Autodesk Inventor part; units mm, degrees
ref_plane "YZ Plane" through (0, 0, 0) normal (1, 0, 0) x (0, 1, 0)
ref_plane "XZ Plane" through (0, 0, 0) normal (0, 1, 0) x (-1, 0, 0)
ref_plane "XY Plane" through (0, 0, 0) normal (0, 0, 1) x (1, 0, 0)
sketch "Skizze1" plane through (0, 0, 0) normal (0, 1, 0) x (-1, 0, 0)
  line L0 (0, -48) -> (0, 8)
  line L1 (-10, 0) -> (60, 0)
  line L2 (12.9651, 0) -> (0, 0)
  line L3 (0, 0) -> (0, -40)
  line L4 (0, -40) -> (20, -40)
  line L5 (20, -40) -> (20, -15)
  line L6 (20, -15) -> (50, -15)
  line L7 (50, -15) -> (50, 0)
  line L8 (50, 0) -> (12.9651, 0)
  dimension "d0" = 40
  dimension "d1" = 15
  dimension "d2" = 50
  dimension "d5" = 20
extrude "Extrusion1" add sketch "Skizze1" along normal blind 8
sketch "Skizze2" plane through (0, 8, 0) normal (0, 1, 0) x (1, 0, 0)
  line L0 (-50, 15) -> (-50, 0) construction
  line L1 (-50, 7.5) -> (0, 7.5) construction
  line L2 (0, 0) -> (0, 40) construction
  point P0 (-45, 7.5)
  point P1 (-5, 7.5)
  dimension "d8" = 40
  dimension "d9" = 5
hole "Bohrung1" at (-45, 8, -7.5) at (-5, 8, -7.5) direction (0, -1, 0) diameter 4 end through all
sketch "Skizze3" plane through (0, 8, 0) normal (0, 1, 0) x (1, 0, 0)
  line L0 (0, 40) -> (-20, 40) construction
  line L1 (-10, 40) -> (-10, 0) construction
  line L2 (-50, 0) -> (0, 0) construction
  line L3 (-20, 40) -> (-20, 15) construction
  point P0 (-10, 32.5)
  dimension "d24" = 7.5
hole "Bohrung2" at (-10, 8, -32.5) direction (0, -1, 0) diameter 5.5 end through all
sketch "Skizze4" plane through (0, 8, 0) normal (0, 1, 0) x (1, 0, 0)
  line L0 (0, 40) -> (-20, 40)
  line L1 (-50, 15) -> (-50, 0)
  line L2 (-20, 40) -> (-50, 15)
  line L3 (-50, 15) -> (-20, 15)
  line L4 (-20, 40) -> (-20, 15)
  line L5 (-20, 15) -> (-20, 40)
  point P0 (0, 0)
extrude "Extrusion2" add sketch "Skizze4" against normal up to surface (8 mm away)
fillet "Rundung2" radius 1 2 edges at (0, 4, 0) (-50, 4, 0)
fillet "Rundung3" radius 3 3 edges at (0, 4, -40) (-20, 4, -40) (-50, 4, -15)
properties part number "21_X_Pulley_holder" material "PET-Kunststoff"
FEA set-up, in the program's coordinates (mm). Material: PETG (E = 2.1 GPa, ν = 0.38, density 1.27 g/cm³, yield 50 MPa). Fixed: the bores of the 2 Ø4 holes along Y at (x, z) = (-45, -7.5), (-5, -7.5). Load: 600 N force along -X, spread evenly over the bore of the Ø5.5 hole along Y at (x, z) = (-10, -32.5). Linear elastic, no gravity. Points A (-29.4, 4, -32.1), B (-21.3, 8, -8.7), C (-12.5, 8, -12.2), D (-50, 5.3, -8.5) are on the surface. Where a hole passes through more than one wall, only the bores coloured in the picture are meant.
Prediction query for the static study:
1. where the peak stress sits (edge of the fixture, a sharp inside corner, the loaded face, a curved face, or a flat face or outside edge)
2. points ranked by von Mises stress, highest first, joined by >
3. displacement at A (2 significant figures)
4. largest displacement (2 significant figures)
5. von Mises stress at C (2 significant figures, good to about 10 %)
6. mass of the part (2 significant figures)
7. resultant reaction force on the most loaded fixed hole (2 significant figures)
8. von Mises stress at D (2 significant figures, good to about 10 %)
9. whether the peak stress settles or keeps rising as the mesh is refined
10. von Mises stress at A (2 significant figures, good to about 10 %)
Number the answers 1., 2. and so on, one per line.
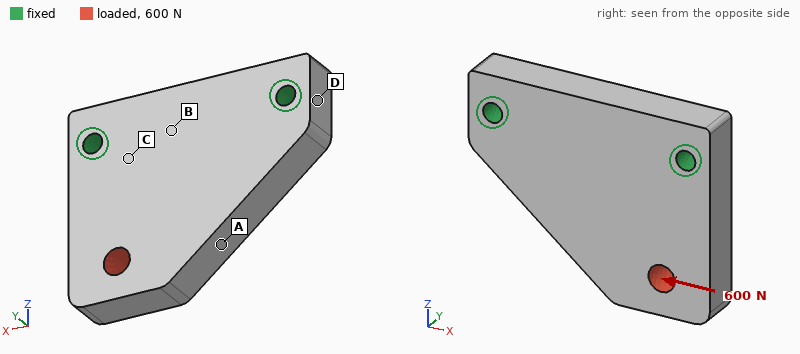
1. edge of the fixture
2. A > D > C > B
3. 0.083 mm
4. 0.14 mm
5. 2.6 MPa
6. 16 g
7. 500 N
8. 4.1 MPa
9. keeps rising
10. 5.4 MPa
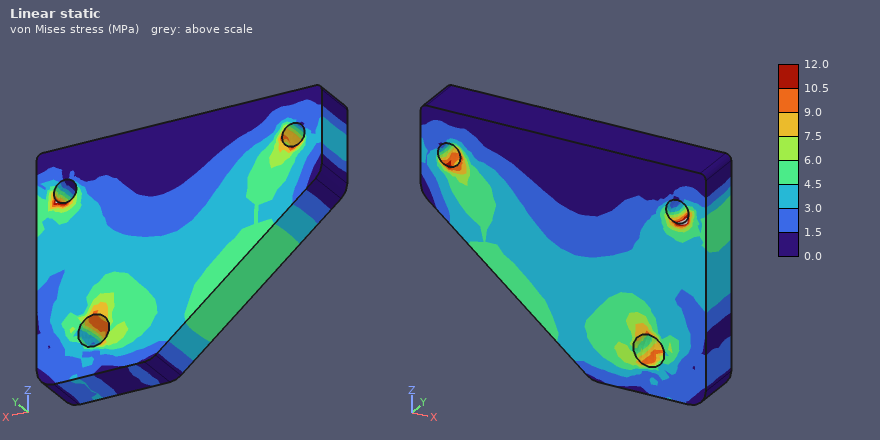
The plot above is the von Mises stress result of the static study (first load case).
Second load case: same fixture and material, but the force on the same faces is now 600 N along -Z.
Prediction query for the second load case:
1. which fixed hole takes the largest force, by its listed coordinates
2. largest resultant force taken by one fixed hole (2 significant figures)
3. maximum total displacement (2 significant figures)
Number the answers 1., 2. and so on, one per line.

1. (-5, -7.5)
2. 530 N
3. 76 µm
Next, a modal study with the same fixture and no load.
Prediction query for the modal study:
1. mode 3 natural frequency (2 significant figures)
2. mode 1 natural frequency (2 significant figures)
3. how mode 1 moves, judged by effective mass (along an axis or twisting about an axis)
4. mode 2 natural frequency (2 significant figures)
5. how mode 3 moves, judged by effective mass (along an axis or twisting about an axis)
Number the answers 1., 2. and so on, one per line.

1. 5400 Hz
2. 1500 Hz
3. along Y
4. 3700 Hz
5. along X
